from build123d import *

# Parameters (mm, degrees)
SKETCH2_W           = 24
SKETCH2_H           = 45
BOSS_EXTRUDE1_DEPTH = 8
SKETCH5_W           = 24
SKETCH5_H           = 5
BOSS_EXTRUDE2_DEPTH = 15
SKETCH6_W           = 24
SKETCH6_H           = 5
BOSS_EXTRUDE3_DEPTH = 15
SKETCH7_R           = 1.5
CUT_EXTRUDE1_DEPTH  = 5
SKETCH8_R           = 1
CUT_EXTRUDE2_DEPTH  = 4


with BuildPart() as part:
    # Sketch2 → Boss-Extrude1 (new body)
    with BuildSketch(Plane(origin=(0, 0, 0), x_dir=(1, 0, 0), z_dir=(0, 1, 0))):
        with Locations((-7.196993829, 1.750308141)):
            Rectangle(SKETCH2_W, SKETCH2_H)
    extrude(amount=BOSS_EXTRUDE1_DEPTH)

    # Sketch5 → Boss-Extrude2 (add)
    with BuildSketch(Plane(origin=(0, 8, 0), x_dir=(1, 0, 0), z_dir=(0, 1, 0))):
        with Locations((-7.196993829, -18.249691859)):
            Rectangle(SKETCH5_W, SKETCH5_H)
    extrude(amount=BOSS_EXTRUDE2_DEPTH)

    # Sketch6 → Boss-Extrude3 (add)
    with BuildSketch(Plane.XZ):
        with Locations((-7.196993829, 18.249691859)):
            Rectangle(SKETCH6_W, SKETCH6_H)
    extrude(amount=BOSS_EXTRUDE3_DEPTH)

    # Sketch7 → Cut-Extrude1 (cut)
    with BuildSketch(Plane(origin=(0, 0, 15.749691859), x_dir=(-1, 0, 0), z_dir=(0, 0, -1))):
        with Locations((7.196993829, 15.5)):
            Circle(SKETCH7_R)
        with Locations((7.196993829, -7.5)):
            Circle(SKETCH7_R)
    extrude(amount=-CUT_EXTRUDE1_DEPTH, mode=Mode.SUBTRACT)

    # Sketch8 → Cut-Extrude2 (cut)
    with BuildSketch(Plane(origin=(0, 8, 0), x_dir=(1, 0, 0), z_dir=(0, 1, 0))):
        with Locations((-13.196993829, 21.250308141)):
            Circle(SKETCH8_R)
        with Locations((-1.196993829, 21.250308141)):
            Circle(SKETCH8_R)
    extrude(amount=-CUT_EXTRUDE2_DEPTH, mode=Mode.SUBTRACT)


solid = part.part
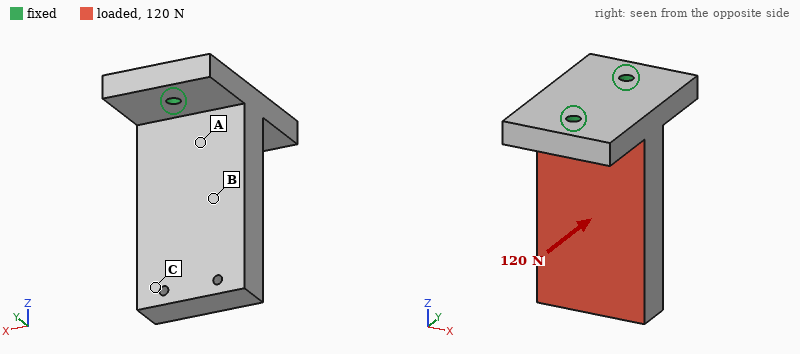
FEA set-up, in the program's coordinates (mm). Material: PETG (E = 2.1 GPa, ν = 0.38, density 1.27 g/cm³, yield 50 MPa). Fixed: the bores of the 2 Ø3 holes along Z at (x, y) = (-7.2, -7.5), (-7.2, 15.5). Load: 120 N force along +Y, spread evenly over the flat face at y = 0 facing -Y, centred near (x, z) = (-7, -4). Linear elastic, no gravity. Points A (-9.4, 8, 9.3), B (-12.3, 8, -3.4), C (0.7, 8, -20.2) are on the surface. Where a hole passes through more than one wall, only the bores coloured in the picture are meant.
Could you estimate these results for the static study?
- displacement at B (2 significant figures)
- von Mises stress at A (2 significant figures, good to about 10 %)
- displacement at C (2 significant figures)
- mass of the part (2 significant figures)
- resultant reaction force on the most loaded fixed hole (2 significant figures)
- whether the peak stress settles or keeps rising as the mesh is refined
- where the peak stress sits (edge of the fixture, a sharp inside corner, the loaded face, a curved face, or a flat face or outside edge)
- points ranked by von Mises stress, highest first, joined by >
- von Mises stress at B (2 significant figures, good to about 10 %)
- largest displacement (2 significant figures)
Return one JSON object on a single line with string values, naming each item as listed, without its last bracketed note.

{"displacement at B": "0.32 mm", "von Mises stress at A": "6.1 MPa", "displacement at C": "0.67 mm", "mass of the part": "15 g", "resultant reaction force on the most loaded fixed hole": "150 N", "whether the peak stress settles or keeps rising as the mesh is refined": "keeps rising", "where the peak stress sits": "edge of the fixture", "points ranked by von Mises stress, highest first, joined by >": "A > B > C", "von Mises stress at B": "2.6 MPa", "largest displacement": "0.76 mm"}
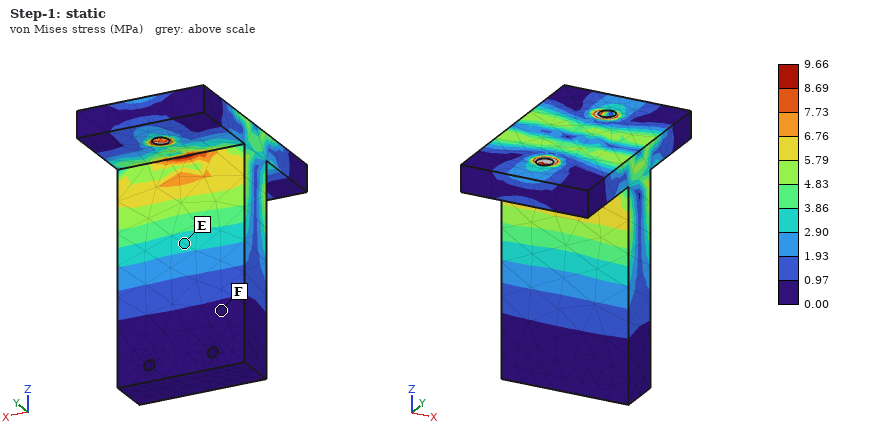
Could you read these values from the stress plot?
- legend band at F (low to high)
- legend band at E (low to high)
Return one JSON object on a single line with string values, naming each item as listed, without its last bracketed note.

{"legend band at F": "0.00 to 0.97 MPa", "legend band at E": "2.90 to 3.86 MPa"}
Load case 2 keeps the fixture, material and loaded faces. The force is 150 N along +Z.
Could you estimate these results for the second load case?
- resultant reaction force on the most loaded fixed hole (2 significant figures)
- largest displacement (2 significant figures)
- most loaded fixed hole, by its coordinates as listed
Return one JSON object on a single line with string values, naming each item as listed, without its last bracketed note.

{"resultant reaction force on the most loaded fixed hole": "110 N", "largest displacement": "0.22 mm", "most loaded fixed hole, by its coordinates as listed": "(-7.2, -7.5)"}
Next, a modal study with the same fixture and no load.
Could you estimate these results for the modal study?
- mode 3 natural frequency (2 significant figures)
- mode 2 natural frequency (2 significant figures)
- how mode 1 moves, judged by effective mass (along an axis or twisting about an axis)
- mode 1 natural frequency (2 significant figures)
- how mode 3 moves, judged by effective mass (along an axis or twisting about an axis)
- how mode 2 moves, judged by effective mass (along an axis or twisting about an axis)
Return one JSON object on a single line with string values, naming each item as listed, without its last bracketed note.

{"mode 3 natural frequency": "2700 Hz", "mode 2 natural frequency": "800 Hz", "how mode 1 moves, judged by effective mass": "along X", "mode 1 natural frequency": "730 Hz", "how mode 3 moves, judged by effective mass": "twisting about Z", "how mode 2 moves, judged by effective mass": "along Y"}
